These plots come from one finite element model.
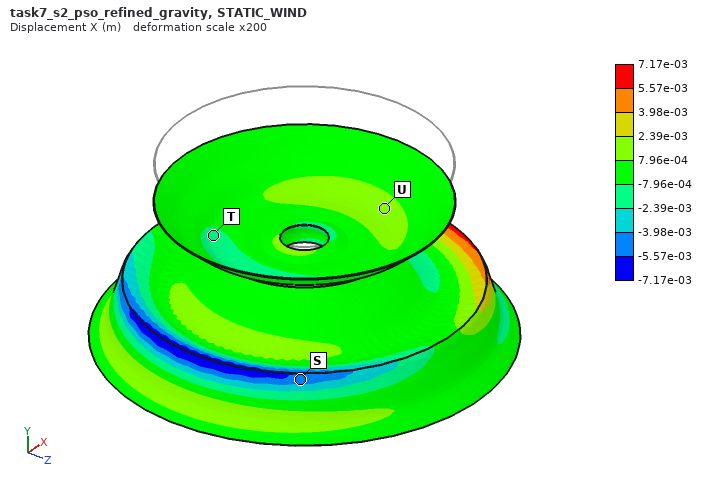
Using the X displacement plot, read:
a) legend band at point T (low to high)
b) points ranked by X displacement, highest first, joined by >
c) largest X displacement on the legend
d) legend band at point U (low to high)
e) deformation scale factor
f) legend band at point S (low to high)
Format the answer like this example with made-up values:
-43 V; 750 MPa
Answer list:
-2.39e-03 to -7.96e-04 m; U > T > S; 7.17e-03 m; 7.96e-04 to 2.39e-03 m; 200; -5.57e-03 to -3.98e-03 m
